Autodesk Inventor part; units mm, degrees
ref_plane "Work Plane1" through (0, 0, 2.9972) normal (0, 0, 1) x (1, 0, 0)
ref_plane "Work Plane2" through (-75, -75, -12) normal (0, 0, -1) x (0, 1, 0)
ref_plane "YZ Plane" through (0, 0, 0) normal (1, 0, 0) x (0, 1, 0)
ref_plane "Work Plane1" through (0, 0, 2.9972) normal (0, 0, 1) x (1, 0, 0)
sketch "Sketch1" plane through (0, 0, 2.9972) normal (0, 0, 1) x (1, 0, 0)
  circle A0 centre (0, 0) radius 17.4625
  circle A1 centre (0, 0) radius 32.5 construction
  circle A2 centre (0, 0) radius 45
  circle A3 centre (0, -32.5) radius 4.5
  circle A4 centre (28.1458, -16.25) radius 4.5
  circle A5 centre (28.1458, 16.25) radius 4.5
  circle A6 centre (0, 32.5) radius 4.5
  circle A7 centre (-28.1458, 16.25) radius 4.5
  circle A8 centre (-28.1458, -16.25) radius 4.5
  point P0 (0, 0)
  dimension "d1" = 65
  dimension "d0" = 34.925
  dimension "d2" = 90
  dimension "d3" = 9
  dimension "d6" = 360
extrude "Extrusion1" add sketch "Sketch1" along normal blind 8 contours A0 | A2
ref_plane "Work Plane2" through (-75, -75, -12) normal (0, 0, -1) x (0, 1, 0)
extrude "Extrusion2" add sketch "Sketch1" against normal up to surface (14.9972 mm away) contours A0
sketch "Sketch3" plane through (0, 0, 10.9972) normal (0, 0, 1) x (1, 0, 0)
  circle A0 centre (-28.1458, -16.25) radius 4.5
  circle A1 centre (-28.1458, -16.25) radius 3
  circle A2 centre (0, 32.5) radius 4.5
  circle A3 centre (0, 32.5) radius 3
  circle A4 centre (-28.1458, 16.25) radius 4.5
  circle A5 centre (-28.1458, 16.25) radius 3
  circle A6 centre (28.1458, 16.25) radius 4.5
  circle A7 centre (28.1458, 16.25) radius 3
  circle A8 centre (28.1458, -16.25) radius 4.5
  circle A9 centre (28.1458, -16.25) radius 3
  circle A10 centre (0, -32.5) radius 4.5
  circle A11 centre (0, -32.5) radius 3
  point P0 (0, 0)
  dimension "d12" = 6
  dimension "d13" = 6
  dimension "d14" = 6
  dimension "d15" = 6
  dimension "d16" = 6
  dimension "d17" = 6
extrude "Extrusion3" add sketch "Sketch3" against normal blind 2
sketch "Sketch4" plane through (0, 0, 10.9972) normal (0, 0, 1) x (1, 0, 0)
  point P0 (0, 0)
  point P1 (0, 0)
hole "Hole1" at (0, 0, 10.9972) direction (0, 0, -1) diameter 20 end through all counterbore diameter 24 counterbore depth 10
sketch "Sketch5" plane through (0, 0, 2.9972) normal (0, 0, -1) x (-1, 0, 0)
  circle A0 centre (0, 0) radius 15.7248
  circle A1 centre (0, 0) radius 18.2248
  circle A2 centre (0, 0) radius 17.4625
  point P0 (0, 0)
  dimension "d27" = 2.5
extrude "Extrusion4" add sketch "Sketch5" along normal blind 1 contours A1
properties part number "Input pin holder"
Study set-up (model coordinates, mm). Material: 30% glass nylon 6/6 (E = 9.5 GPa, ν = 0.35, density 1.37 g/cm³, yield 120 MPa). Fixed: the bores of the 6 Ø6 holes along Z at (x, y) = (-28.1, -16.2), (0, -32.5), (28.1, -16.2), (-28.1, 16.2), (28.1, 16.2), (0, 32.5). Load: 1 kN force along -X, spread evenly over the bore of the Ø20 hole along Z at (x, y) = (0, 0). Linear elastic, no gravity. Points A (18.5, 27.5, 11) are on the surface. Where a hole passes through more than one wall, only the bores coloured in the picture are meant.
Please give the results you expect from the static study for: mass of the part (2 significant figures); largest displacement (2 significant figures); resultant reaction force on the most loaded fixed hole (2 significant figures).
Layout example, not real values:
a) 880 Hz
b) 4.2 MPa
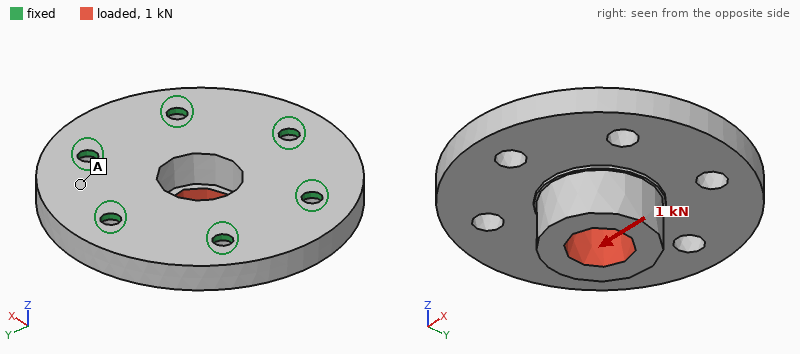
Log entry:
a) 74 g
b) 26 µm
c) 270 N
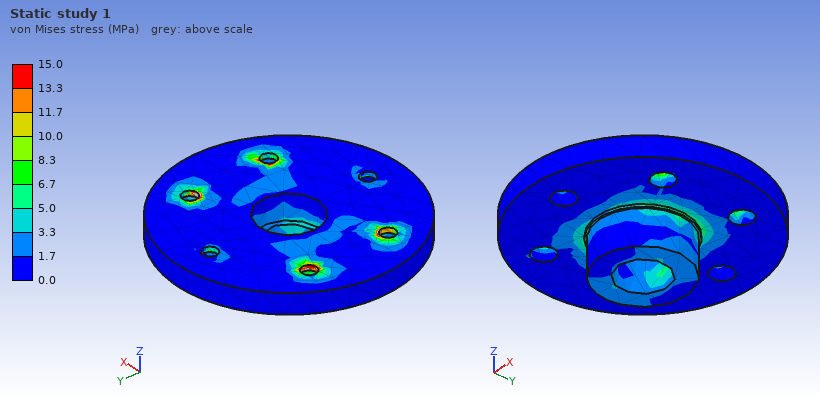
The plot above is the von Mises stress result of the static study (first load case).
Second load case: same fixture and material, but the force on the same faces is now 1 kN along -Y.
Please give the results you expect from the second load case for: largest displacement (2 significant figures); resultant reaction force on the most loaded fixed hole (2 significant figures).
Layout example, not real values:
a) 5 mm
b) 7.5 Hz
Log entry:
a) 26 µm
b) 300 N
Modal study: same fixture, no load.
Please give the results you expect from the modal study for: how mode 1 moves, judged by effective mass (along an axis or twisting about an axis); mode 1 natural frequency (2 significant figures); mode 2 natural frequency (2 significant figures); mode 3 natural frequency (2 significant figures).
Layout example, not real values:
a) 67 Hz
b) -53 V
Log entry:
a) along Z
b) 6100 Hz
c) 7300 Hz
d) 7300 Hz
